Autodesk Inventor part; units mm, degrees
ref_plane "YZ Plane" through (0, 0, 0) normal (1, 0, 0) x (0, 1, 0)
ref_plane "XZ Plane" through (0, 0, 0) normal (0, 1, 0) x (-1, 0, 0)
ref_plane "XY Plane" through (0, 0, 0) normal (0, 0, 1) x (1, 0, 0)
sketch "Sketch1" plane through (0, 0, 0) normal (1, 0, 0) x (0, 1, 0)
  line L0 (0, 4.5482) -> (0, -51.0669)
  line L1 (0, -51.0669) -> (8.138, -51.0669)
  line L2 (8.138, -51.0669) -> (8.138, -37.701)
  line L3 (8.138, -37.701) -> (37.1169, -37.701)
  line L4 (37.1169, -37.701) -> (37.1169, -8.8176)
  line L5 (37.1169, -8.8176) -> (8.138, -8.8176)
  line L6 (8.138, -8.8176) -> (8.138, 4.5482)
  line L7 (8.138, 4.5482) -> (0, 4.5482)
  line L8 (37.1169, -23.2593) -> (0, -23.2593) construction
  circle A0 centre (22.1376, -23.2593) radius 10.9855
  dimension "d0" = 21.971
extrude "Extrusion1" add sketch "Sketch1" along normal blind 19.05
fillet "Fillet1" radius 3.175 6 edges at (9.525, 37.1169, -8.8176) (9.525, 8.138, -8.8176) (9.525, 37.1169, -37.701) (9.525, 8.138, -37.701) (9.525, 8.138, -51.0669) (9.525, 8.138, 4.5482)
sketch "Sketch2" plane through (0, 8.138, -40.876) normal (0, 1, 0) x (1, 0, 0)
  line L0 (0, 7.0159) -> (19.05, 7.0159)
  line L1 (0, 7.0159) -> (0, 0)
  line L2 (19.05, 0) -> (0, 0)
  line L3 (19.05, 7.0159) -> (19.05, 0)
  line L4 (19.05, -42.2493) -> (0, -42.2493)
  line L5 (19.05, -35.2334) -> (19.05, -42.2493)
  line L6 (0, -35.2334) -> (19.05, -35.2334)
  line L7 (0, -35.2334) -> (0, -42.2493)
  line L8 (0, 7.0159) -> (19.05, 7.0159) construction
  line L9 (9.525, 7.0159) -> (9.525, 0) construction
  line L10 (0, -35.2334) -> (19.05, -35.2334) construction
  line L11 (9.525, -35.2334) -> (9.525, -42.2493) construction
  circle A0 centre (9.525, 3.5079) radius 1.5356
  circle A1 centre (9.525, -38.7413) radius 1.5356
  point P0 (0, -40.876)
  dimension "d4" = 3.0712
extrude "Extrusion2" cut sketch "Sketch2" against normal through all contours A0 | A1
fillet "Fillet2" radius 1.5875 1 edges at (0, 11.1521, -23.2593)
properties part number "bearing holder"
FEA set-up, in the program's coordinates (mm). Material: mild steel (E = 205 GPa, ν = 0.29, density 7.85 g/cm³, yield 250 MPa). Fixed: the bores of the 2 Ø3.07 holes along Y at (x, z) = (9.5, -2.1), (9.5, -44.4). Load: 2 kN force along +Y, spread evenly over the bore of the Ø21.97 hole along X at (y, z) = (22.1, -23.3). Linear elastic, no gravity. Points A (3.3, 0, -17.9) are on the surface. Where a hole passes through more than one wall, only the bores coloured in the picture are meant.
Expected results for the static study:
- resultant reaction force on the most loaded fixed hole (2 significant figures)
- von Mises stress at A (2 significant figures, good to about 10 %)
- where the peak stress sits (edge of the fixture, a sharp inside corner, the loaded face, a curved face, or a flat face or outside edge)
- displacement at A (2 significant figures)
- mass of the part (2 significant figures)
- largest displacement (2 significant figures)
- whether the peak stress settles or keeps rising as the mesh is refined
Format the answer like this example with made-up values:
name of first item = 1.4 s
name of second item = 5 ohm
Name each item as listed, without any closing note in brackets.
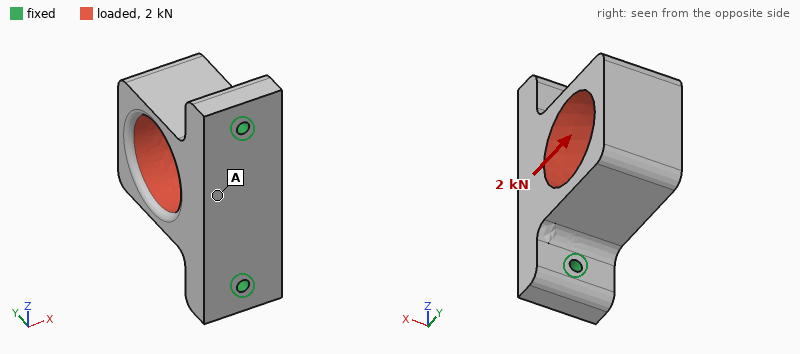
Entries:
resultant reaction force on the most loaded fixed hole = 1.1 kN
von Mises stress at A = 7.7 MPa
where the peak stress sits = edge of the fixture
displacement at A = 2.0 µm
mass of the part = 130 g
largest displacement = 4.6 µm
whether the peak stress settles or keeps rising as the mesh is refined = keeps rising
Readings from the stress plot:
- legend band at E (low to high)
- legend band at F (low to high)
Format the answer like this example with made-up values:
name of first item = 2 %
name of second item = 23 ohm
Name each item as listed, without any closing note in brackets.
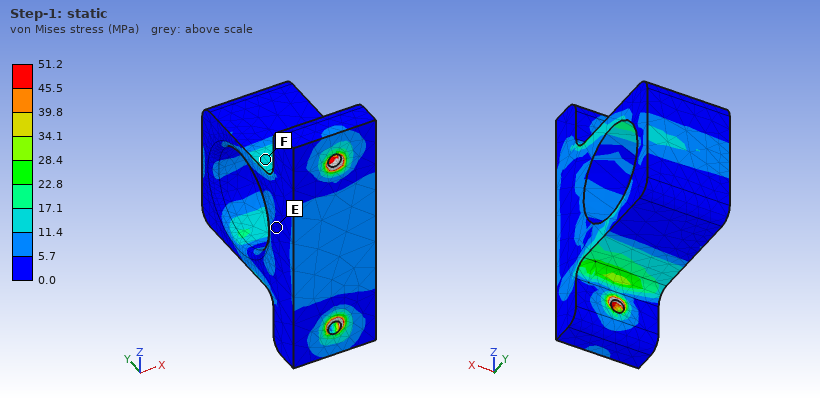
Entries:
legend band at E = 0.0 to 5.7 MPa
legend band at F = 11.4 to 17.1 MPa
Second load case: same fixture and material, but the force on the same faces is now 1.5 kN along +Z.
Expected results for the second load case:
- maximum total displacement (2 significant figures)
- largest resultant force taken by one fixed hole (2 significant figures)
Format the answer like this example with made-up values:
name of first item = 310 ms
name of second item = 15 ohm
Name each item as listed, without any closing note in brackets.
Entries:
maximum total displacement = 11 µm
largest resultant force taken by one fixed hole = 1.0 kN
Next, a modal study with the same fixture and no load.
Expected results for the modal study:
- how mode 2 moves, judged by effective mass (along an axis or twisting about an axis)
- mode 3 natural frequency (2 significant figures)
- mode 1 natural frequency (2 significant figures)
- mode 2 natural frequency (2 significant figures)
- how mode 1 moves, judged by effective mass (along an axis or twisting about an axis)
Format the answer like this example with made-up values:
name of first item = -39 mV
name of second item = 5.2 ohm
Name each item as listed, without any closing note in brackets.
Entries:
how mode 2 moves, judged by effective mass = along Z
mode 3 natural frequency = 12 kHz
mode 1 natural frequency = 4900 Hz
mode 2 natural frequency = 7600 Hz
how mode 1 moves, judged by effective mass = along X
